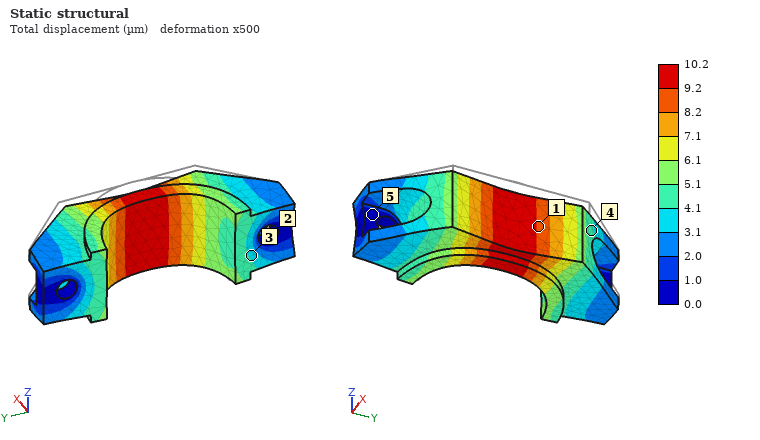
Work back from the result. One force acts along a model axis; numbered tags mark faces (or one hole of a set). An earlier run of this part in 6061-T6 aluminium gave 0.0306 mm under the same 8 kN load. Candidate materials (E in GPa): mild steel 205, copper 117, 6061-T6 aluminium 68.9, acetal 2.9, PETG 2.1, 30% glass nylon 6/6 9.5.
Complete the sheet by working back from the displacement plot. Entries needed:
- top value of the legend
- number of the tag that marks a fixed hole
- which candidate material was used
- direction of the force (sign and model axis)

10.2 µm
2
mild steel
-X
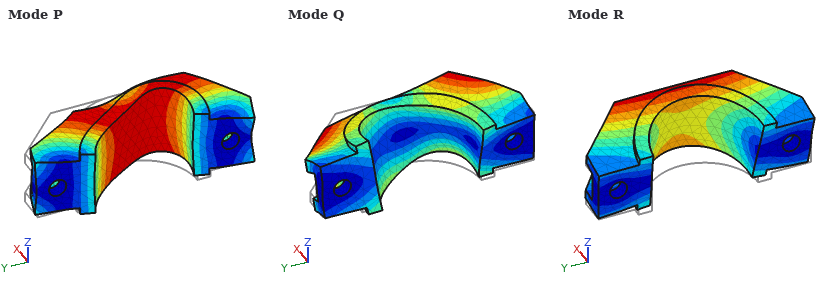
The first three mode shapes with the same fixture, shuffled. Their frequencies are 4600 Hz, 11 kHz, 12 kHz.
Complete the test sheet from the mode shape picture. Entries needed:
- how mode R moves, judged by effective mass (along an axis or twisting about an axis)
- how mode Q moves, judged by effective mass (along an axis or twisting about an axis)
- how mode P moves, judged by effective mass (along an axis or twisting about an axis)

along Z
twisting about X
along Y
